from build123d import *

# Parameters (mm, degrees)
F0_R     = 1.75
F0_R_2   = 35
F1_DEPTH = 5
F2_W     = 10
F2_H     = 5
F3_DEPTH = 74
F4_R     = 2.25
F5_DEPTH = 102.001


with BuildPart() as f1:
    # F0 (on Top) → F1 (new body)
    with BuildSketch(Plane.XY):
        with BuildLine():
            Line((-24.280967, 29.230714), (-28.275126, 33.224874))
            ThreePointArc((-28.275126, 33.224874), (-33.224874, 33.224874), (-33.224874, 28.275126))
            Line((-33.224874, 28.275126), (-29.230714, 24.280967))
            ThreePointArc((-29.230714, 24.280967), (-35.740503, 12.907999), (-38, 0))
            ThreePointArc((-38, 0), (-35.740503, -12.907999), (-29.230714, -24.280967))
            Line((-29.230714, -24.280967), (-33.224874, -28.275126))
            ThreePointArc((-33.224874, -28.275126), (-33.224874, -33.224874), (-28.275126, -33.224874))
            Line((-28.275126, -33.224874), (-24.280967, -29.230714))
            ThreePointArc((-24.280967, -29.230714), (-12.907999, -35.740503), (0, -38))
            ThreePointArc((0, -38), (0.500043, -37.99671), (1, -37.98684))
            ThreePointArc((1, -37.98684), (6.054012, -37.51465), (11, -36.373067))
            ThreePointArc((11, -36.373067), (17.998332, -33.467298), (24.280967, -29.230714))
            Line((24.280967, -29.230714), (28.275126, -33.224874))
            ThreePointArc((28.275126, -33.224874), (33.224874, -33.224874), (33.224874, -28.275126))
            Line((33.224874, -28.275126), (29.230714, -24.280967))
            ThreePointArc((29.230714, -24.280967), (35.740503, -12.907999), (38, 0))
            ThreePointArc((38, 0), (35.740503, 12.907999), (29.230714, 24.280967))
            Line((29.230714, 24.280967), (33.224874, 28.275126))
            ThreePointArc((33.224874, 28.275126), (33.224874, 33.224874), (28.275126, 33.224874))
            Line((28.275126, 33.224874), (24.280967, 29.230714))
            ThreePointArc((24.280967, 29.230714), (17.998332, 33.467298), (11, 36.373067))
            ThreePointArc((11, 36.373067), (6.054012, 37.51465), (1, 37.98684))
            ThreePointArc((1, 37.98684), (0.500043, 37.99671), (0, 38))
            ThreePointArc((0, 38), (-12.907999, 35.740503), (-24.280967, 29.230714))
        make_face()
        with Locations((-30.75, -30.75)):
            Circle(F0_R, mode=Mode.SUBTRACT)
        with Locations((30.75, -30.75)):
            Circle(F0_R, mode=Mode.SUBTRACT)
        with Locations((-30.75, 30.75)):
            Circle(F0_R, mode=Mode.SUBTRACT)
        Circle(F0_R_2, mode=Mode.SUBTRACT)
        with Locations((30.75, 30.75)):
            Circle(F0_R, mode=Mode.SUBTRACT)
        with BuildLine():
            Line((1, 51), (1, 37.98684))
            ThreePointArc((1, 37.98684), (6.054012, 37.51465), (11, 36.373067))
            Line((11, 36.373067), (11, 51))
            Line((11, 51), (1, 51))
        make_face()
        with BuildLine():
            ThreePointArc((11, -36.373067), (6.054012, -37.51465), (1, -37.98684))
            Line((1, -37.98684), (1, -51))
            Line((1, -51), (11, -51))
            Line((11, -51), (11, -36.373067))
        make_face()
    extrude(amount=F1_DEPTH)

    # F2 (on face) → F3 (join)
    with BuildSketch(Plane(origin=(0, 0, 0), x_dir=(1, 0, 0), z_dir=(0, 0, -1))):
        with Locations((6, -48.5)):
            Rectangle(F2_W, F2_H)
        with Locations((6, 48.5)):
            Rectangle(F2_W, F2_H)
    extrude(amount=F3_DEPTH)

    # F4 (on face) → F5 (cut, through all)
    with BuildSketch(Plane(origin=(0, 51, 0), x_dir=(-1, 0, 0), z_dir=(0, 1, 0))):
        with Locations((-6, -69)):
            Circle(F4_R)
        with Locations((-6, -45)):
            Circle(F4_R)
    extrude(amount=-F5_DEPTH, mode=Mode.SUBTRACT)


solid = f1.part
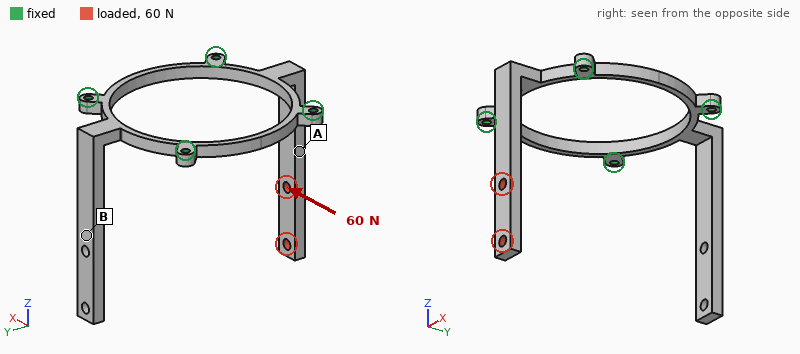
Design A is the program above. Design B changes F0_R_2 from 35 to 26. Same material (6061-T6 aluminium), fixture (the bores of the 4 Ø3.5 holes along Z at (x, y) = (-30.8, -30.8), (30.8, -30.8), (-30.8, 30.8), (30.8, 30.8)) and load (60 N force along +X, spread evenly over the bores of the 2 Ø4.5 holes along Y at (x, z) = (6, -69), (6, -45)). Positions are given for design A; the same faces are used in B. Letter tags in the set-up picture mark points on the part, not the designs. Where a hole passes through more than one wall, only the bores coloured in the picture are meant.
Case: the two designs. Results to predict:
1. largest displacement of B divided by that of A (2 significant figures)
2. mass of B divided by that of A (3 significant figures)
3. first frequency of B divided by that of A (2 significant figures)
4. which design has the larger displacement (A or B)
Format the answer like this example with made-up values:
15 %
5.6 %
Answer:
0.72
1.67
1.7
A
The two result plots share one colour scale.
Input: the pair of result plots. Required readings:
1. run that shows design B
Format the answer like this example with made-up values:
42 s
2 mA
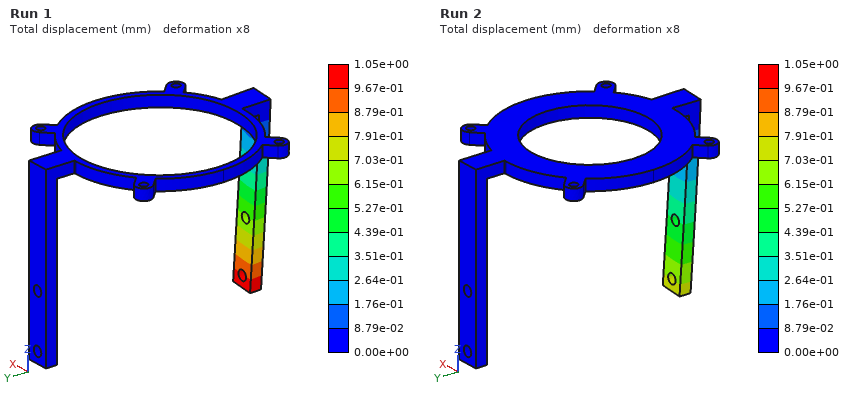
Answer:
Run 2
